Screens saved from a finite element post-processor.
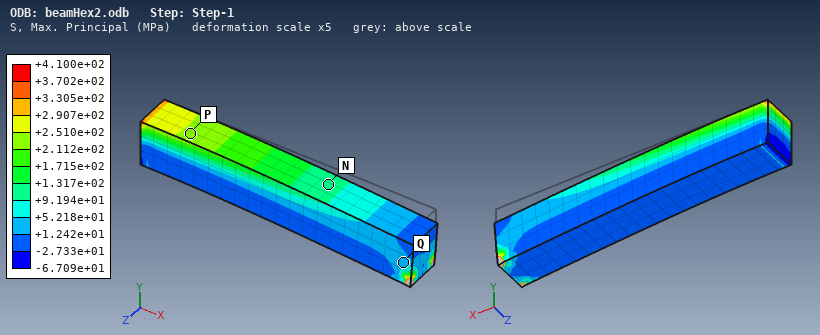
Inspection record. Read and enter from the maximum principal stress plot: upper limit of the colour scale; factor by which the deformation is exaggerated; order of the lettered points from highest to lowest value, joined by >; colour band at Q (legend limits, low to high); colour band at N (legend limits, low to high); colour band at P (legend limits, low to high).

+4.100e+02 MPa
5
P > N > Q
+1.242e+01 to +5.218e+01 MPa
+9.194e+01 to +1.317e+02 MPa
+2.112e+02 to +2.510e+02 MPa
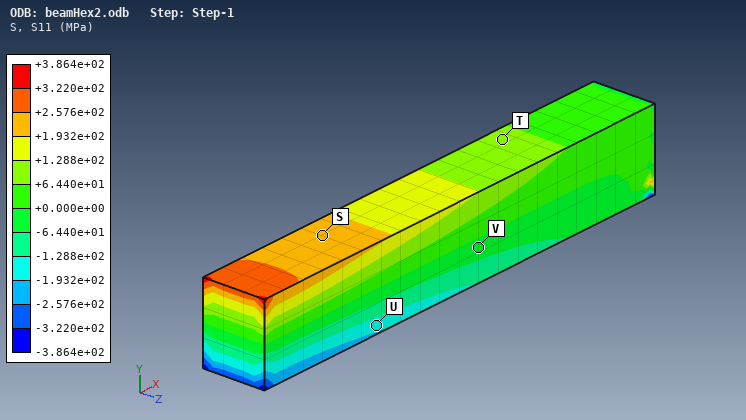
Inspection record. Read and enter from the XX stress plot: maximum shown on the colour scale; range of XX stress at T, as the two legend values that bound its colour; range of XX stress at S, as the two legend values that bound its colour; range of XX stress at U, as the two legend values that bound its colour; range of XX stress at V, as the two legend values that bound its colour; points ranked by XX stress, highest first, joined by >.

+3.864e+02 MPa
+6.440e+01 to +1.288e+02 MPa
+1.932e+02 to +2.576e+02 MPa
-1.932e+02 to -1.288e+02 MPa
-6.440e+01 to +0.000e+00 MPa
S > T > V > U
